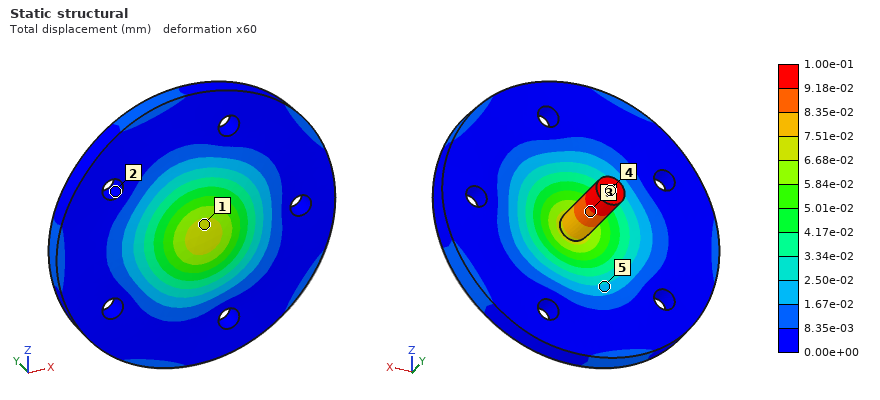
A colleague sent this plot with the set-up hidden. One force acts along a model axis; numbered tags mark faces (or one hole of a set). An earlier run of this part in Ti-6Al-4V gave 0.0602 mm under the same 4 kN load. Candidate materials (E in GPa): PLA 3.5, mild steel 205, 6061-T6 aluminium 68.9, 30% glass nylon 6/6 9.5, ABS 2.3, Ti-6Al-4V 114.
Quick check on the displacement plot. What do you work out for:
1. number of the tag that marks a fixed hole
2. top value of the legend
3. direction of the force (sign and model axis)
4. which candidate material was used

2
1.00e-01 mm
-Y
6061-T6 aluminium
